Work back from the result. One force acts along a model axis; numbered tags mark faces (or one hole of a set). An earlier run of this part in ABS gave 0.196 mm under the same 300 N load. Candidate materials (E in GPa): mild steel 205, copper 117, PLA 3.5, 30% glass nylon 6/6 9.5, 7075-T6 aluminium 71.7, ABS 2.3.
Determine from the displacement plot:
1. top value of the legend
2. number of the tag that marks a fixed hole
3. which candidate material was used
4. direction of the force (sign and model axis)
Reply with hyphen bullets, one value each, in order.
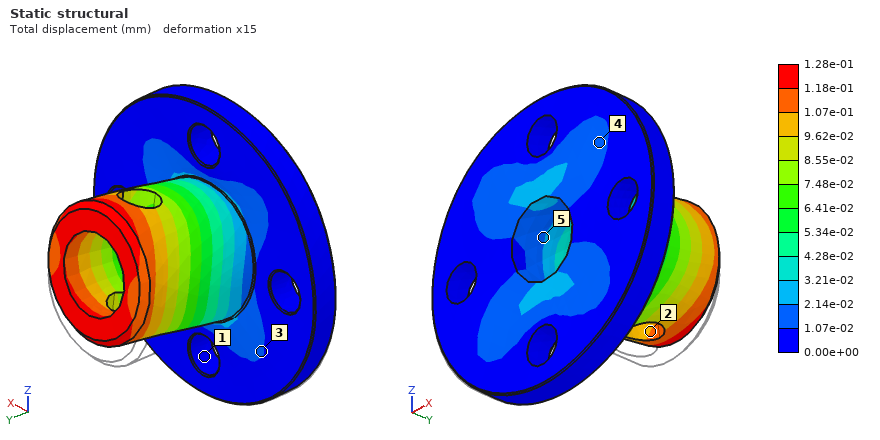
- 1.28e-01 mm
- 1
- PLA
- +Z
